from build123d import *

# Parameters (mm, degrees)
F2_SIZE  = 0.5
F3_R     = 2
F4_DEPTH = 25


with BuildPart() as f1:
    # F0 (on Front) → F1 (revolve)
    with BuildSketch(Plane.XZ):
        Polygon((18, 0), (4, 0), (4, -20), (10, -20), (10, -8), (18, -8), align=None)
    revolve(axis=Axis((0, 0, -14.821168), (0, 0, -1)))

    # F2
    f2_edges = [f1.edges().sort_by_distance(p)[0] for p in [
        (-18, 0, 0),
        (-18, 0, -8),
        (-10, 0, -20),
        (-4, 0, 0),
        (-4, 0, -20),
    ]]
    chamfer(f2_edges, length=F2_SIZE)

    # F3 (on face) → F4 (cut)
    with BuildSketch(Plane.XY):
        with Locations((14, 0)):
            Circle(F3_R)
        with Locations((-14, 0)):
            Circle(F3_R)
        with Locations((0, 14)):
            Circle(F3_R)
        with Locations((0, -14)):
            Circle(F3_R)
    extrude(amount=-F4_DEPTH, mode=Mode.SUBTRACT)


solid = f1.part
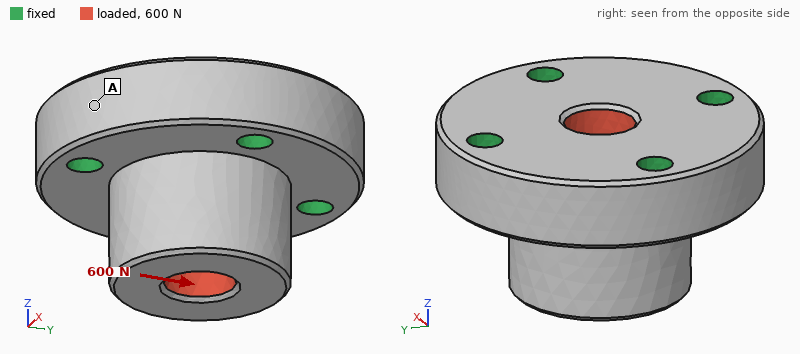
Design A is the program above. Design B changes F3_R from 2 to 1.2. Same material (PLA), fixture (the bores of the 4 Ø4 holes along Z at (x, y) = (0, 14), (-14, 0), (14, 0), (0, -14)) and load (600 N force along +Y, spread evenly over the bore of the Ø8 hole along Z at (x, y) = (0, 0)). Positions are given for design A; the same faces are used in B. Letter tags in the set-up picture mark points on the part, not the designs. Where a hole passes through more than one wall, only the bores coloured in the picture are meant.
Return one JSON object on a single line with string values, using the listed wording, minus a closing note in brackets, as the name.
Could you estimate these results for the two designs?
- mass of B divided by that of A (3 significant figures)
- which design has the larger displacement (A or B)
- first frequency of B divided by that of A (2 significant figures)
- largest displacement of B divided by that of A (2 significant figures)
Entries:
{"mass of B divided by that of A": "1.02", "which design has the larger displacement": "B", "first frequency of B divided by that of A": "0.92", "largest displacement of B divided by that of A": "1.1"}
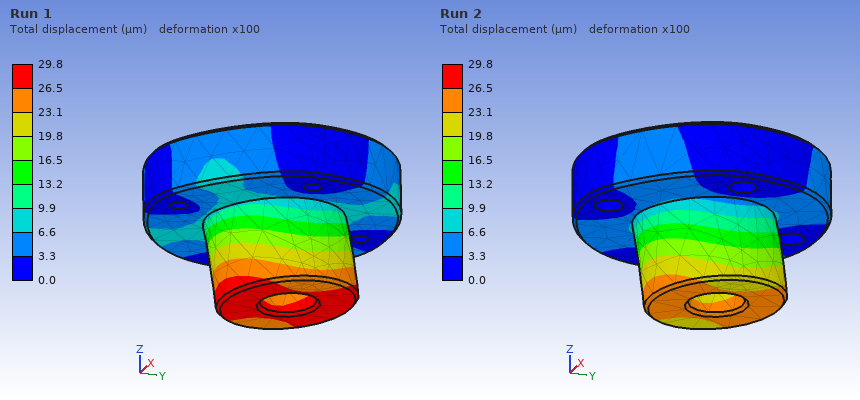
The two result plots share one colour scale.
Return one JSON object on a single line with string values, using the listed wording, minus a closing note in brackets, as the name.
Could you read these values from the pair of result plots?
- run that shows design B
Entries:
{"run that shows design B": "Run 1"}
